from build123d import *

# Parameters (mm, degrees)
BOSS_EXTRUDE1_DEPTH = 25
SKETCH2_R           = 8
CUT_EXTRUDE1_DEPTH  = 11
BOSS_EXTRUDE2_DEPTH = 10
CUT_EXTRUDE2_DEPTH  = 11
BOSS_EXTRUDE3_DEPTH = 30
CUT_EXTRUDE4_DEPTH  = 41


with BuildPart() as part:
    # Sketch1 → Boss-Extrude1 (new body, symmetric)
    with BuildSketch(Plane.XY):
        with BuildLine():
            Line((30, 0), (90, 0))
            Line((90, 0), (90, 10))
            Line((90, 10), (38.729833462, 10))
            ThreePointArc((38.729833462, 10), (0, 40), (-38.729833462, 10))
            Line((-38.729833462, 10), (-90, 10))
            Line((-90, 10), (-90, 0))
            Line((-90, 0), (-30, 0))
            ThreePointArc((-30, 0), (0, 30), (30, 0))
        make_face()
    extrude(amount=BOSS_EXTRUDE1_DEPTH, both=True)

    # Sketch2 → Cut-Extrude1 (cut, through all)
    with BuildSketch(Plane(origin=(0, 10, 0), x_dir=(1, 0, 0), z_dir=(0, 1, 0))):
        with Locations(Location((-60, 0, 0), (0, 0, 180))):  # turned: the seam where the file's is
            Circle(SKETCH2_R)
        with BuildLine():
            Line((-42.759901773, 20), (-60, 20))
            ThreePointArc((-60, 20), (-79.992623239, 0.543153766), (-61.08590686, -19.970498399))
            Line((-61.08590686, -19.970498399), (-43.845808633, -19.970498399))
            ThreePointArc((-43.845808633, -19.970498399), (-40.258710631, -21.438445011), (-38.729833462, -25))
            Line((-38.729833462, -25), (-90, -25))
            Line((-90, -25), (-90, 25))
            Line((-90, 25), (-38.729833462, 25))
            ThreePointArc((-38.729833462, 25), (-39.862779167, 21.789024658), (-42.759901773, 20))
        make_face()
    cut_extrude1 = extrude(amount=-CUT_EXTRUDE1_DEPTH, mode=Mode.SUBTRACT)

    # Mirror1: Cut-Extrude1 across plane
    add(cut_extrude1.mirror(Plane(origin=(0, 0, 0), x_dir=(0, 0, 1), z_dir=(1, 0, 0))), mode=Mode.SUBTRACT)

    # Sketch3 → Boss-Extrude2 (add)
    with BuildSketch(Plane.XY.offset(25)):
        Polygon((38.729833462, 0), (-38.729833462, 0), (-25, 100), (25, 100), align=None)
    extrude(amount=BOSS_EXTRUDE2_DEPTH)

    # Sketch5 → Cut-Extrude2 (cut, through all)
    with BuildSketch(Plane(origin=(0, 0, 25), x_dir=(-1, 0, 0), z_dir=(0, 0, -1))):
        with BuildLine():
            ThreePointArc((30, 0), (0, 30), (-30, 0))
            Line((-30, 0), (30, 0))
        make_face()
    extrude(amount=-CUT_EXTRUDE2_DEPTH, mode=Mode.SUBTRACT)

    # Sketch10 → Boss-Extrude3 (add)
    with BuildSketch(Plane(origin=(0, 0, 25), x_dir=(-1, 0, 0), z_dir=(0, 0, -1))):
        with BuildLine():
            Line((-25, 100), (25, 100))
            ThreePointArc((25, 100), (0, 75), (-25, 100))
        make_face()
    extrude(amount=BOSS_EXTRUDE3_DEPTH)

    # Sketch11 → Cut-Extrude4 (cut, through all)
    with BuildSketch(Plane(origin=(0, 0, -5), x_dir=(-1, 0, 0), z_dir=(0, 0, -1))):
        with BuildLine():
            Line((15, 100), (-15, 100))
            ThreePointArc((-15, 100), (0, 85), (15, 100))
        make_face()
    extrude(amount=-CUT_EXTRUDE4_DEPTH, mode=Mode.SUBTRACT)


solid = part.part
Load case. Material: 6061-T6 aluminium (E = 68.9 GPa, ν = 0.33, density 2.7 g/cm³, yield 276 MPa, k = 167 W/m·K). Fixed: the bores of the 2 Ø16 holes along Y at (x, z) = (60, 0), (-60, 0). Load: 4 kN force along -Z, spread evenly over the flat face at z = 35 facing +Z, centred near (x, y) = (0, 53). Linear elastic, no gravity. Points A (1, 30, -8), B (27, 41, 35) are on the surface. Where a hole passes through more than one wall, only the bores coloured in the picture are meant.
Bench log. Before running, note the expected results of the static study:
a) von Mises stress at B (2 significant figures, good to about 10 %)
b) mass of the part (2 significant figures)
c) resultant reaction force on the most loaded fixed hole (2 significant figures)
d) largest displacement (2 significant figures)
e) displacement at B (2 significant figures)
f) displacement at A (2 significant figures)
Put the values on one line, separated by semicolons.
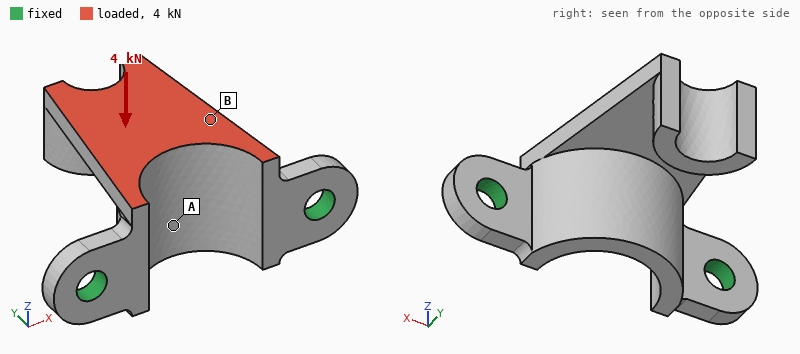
55 MPa; 390 g; 2.1 kN; 0.81 mm; 0.27 mm; 0.14 mm
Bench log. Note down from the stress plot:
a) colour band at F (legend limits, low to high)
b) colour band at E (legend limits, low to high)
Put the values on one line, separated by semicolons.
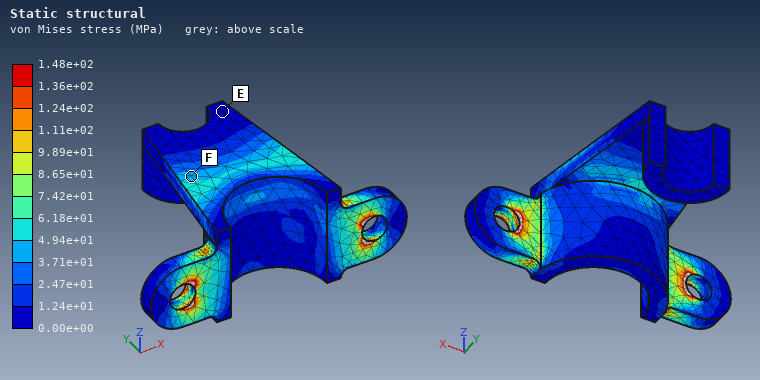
3.71e+01 to 4.94e+01 MPa; 0.00e+00 to 1.24e+01 MPa
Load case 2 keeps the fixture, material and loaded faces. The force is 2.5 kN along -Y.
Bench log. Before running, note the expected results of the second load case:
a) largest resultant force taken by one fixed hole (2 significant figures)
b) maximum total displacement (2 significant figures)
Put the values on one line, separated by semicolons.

1.5 kN; 0.27 mm
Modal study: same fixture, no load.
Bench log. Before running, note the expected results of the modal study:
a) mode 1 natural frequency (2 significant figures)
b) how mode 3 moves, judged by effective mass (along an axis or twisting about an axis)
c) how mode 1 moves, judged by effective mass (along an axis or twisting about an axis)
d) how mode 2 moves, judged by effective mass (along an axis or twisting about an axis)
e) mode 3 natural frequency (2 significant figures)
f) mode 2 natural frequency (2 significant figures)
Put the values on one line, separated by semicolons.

840 Hz; along Y; along Z; along X; 2100 Hz; 1900 Hz
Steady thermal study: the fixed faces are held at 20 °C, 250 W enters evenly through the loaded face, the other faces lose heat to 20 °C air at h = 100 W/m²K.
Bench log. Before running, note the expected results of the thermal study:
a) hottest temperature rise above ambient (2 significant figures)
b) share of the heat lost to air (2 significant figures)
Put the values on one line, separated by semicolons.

81 K; 49 %
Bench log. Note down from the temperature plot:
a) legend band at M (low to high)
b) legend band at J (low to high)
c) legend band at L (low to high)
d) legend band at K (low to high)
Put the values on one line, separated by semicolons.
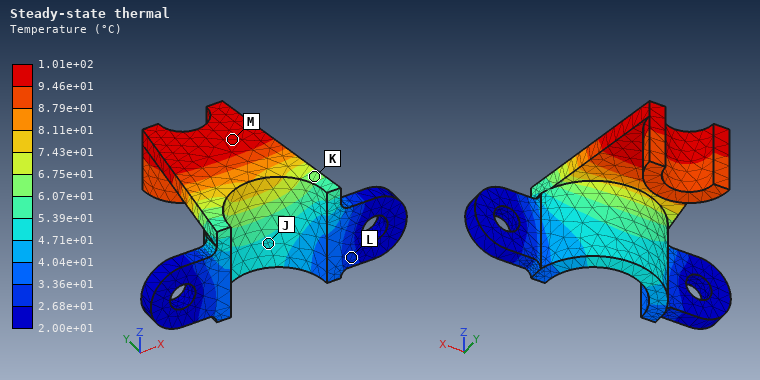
9.46e+01 to 1.01e+02 °C; 4.71e+01 to 5.39e+01 °C; 2.68e+01 to 3.36e+01 °C; 6.07e+01 to 6.75e+01 °C
